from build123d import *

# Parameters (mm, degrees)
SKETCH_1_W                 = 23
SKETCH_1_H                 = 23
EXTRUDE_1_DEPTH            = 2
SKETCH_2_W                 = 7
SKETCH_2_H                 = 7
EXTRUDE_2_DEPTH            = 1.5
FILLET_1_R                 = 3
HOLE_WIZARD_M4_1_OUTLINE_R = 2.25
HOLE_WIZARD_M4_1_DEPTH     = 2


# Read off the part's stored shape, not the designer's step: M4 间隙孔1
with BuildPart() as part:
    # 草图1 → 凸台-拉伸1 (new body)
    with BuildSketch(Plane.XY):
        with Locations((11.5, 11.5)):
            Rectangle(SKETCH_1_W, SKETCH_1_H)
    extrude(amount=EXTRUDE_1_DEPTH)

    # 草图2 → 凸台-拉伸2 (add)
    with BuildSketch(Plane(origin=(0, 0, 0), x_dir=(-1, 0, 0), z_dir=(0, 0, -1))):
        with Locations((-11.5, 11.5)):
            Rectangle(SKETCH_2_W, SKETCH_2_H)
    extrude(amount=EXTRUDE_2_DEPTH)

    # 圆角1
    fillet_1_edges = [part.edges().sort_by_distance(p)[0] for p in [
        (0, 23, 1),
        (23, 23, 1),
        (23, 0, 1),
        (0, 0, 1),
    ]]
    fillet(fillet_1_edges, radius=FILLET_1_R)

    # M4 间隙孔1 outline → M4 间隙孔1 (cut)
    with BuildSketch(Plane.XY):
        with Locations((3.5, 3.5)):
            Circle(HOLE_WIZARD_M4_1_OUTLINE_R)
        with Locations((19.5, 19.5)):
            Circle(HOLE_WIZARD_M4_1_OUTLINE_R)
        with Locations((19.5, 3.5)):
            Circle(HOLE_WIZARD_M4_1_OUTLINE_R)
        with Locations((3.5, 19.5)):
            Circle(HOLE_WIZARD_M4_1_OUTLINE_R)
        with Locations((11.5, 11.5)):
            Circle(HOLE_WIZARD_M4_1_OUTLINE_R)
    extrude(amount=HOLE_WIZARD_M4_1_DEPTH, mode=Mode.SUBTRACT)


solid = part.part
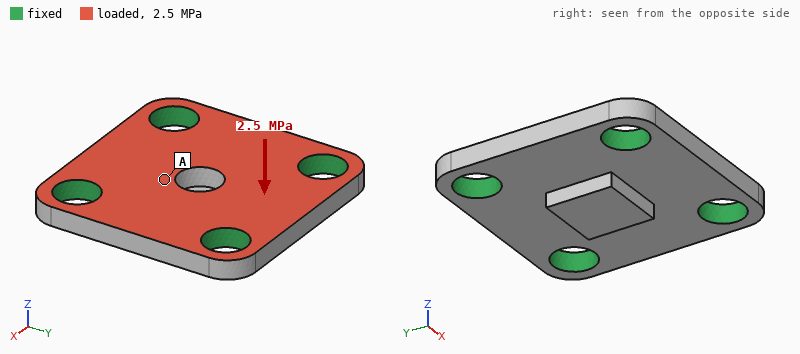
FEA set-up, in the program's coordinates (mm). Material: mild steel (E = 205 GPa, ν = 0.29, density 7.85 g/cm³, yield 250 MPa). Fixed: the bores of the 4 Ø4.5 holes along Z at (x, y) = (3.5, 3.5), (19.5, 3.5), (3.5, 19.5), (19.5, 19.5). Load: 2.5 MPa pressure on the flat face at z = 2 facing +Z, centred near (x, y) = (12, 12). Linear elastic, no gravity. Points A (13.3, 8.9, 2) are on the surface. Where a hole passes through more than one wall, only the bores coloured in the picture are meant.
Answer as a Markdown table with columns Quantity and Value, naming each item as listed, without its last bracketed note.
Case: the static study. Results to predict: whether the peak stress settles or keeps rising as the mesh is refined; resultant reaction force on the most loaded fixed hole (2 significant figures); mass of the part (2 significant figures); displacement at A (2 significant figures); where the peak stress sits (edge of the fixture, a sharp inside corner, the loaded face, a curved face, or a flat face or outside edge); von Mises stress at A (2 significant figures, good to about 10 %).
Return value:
| Quantity | Value |
|---|---|
| whether the peak stress settles or keeps rising as the mesh is refined | keeps rising |
| resultant reaction force on the most loaded fixed hole | 280 N |
| mass of the part | 7.5 g |
| displacement at A | 2.3 µm |
| where the peak stress sits | edge of the fixture |
| von Mises stress at A | 10 MPa |
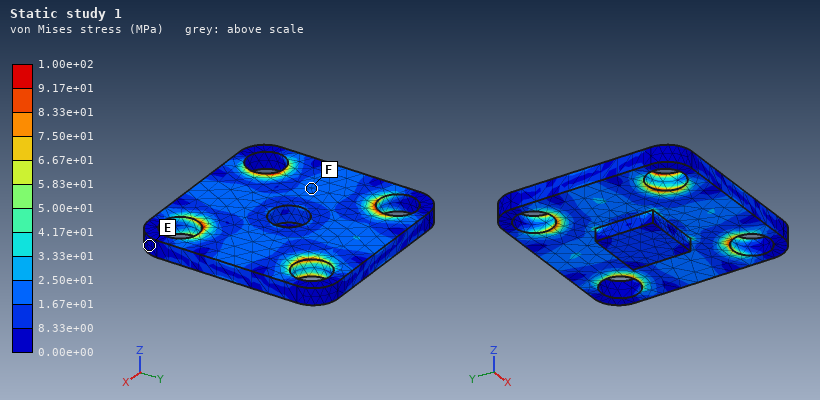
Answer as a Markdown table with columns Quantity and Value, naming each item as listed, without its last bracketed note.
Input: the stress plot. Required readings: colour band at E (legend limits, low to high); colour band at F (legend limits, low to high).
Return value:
| Quantity | Value |
|---|---|
| colour band at E | 0.00e+00 to 8.33e+00 MPa |
| colour band at F | 1.67e+01 to 2.50e+01 MPa |
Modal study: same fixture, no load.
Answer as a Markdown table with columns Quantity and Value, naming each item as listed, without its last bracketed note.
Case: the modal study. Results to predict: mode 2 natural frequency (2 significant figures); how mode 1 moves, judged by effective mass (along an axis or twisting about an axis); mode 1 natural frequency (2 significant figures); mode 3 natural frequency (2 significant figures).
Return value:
| Quantity | Value |
|---|---|
| mode 2 natural frequency | 60 kHz |
| how mode 1 moves, judged by effective mass | along Z |
| mode 1 natural frequency | 41 kHz |
| mode 3 natural frequency | 60 kHz |
